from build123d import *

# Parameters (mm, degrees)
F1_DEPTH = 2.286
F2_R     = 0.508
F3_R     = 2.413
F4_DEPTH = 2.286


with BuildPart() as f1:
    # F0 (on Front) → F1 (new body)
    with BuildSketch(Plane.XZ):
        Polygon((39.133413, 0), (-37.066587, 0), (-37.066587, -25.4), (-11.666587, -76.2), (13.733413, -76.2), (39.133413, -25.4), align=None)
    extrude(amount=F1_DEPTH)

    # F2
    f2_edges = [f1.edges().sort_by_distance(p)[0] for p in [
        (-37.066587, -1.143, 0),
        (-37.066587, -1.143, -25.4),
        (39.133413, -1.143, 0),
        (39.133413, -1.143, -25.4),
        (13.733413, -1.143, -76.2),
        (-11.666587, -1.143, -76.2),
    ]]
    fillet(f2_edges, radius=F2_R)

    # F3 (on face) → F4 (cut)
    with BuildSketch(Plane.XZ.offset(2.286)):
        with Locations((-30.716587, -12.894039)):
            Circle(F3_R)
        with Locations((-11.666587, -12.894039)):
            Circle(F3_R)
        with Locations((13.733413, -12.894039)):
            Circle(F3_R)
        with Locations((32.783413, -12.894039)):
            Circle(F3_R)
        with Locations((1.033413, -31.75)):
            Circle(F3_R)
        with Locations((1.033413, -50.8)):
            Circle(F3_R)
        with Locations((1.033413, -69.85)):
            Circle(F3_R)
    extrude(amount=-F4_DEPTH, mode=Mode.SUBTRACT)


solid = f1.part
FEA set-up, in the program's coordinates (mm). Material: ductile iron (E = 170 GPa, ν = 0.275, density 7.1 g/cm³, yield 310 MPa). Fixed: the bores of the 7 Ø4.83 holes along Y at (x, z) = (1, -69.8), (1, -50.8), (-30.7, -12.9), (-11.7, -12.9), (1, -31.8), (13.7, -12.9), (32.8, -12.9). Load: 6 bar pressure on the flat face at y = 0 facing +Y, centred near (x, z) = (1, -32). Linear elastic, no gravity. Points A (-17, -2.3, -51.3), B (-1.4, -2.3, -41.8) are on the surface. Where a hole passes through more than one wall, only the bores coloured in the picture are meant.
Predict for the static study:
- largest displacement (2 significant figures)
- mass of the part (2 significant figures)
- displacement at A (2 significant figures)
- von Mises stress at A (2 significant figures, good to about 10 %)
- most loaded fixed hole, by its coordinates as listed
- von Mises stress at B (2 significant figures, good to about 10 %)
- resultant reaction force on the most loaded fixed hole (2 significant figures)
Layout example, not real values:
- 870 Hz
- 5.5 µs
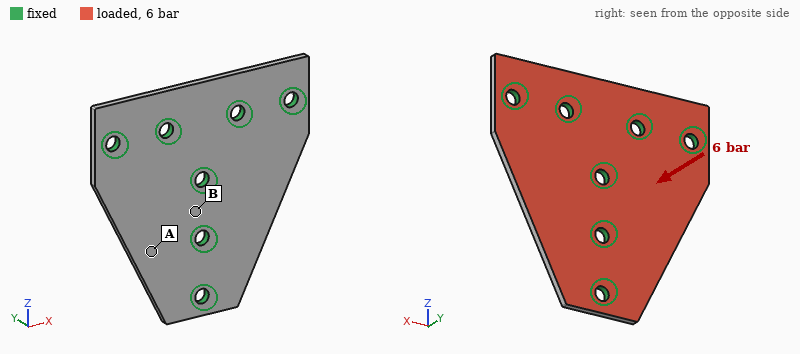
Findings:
- 95 µm
- 71 g
- 57 µm
- 22 MPa
- (1, -50.8)
- 77 MPa
- 570 N
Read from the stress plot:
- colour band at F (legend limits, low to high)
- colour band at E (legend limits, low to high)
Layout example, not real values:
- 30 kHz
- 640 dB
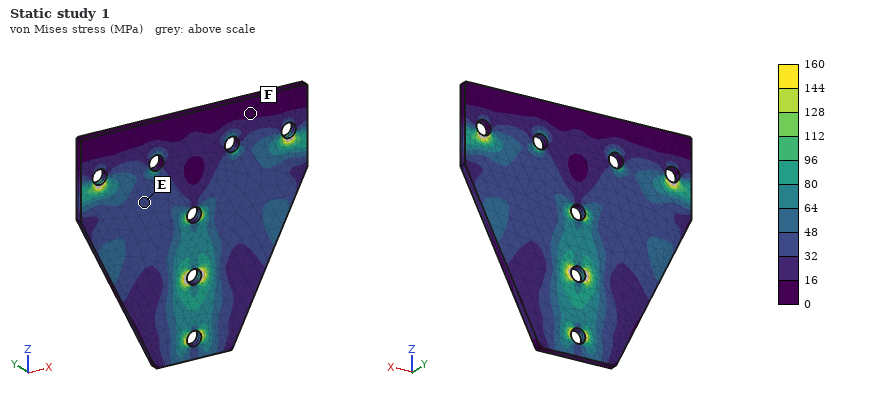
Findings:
- 0 to 16 MPa
- 32 to 48 MPa
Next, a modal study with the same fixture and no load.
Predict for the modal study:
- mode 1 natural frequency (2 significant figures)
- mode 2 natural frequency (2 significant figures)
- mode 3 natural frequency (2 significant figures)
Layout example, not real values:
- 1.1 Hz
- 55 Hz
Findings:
- 4200 Hz
- 4300 Hz
- 8100 Hz
